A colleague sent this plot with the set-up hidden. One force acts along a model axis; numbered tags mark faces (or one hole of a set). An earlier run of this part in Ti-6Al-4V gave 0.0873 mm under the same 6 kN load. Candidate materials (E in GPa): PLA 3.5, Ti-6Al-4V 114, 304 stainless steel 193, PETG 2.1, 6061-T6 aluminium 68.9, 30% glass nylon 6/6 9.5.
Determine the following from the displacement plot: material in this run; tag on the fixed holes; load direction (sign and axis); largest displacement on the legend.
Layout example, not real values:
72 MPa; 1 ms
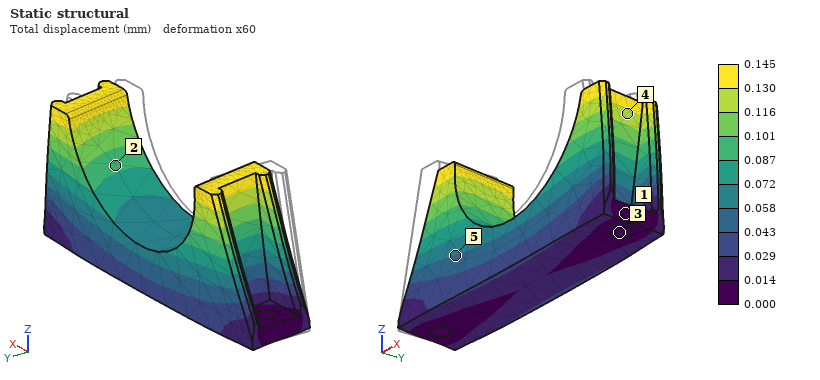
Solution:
6061-T6 aluminium; 3; +Y; 0.145 mm
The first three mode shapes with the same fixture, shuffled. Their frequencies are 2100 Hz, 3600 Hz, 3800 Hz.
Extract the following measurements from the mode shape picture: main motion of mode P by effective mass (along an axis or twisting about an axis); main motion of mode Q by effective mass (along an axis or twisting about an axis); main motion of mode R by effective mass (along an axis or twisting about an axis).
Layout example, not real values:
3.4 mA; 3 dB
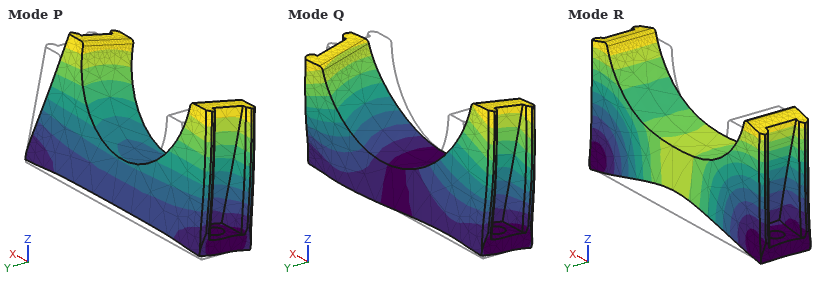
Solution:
along Y; twisting about Z; along Z
